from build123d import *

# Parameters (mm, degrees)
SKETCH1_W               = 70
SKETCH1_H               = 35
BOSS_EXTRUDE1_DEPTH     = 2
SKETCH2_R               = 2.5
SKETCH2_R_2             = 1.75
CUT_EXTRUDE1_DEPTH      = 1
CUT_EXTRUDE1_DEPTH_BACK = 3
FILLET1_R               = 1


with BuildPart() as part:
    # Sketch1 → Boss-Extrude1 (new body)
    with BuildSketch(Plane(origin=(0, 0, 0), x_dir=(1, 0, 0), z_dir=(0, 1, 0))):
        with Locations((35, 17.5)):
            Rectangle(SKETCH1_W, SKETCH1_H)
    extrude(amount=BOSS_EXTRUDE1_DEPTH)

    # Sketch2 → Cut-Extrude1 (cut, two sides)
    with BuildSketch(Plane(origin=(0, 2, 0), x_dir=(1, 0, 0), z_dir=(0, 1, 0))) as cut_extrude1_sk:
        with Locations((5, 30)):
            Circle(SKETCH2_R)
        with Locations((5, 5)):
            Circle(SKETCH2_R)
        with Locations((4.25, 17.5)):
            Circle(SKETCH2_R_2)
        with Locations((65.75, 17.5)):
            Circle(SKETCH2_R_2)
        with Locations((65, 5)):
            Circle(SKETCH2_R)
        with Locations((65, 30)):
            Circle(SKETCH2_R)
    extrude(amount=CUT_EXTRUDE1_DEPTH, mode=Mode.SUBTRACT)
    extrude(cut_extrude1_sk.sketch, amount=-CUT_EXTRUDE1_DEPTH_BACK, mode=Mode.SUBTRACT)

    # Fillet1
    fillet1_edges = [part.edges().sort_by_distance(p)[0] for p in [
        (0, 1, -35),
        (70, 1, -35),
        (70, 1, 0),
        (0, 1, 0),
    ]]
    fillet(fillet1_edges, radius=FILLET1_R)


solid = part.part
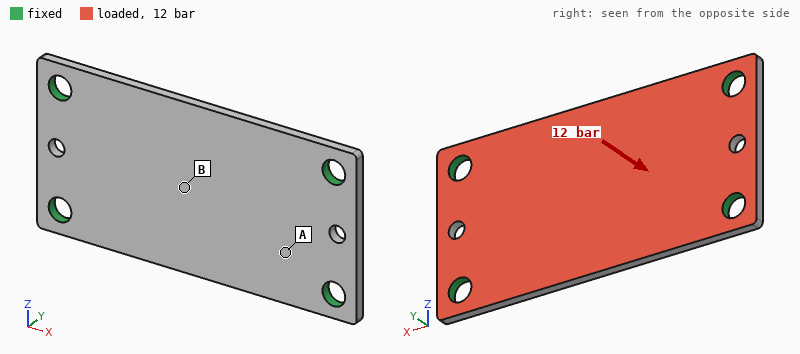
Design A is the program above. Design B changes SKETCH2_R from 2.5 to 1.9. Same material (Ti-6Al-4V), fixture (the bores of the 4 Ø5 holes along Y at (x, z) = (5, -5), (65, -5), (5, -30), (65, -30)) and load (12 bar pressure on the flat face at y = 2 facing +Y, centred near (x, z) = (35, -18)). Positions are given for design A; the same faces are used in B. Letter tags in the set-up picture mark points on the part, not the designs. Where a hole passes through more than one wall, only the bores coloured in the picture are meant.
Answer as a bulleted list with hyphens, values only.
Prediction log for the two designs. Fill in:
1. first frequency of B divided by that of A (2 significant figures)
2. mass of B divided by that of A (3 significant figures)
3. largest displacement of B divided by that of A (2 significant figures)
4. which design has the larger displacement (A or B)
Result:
- 0.95
- 1.01
- 1.1
- B
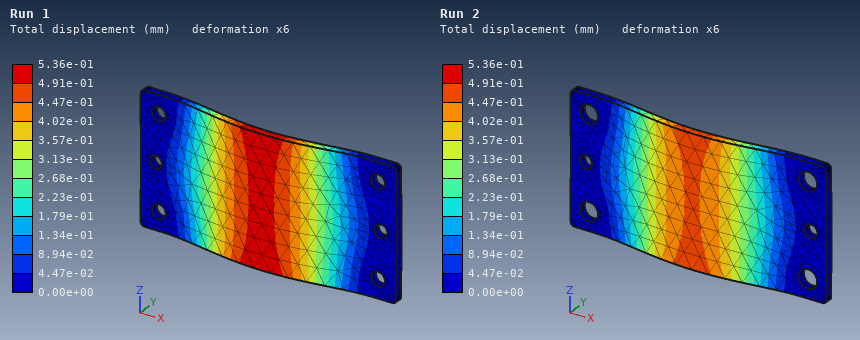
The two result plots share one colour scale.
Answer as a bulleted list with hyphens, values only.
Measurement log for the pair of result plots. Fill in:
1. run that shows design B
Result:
- Run 1
